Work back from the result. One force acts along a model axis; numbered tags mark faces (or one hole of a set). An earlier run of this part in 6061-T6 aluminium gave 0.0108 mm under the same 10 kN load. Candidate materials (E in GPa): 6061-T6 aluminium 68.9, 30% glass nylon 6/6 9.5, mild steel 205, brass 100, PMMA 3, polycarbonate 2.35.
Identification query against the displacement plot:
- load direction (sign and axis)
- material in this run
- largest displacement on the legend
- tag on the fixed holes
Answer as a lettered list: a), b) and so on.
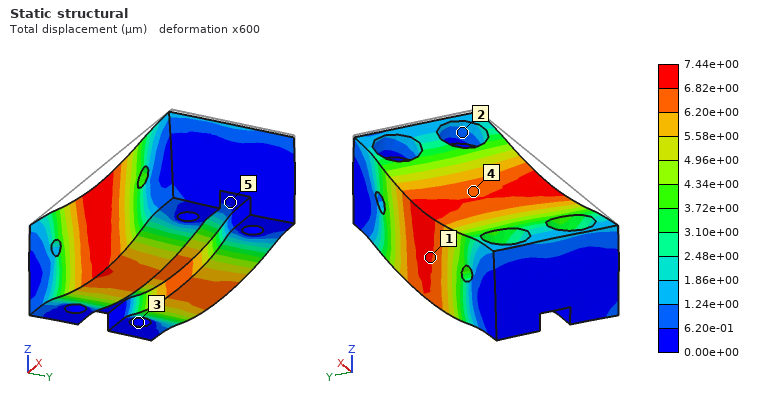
a) -Z
b) brass
c) 7.44e+00 µm
d) 3
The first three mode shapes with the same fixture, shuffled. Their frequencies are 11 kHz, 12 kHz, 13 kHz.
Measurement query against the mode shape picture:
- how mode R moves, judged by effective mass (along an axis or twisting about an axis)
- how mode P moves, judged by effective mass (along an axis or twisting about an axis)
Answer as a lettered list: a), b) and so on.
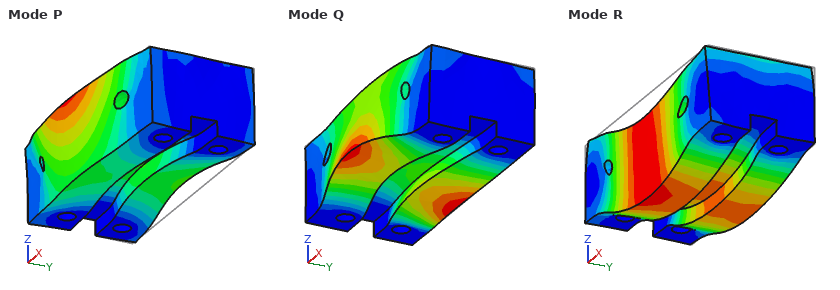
a) along Z
b) along Y
